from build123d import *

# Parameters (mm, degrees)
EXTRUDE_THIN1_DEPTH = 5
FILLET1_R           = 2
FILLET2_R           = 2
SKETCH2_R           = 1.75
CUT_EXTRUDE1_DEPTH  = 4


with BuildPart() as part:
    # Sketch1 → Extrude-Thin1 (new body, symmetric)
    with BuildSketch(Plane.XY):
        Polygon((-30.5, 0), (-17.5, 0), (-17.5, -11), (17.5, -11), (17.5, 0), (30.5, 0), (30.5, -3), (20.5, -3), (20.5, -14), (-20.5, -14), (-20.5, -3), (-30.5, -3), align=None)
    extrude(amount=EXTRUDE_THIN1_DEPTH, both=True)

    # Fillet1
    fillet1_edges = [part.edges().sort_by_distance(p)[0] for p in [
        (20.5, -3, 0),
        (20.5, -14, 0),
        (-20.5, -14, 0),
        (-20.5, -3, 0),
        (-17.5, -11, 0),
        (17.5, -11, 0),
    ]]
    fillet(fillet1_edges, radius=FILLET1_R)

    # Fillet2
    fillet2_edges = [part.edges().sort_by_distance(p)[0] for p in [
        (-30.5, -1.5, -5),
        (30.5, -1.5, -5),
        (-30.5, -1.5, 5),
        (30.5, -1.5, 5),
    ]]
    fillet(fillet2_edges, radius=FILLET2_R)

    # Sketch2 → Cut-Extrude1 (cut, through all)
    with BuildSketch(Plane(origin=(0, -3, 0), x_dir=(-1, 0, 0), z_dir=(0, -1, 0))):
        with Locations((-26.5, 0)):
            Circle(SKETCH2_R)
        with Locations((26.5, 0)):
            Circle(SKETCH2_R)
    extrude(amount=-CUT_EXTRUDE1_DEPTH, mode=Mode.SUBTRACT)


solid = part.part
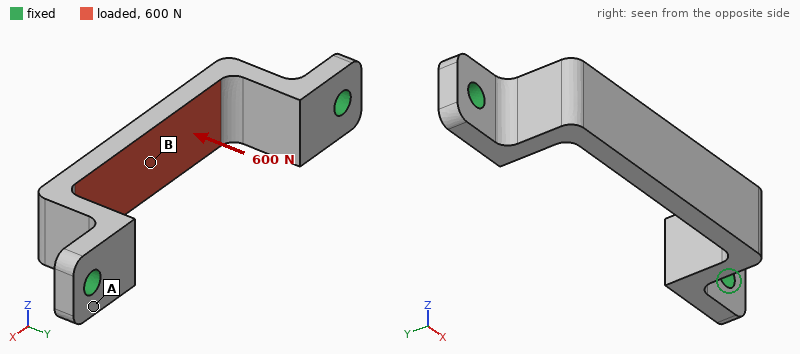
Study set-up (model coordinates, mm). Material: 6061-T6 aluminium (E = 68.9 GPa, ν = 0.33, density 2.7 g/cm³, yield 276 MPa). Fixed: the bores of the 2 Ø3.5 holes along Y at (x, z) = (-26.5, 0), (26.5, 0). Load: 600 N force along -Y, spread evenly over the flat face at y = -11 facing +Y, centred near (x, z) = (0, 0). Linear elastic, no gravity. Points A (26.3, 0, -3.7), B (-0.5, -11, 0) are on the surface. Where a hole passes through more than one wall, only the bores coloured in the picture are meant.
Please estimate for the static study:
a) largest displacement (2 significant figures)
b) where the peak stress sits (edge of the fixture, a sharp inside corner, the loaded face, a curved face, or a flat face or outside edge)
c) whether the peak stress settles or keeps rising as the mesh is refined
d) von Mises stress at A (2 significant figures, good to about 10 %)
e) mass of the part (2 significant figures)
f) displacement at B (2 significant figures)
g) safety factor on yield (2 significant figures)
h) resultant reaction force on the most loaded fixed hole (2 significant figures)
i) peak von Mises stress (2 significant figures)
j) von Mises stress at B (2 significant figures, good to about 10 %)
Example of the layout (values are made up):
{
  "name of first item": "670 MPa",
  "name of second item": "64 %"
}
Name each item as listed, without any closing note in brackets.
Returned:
{
  "largest displacement": "83 µm",
  "where the peak stress sits": "a curved face",
  "whether the peak stress settles or keeps rising as the mesh is refined": "settles",
  "von Mises stress at A": "18 MPa",
  "mass of the part": "6.6 g",
  "displacement at B": "80 µm",
  "safety factor on yield": "2.1",
  "resultant reaction force on the most loaded fixed hole": "430 N",
  "peak von Mises stress": "130 MPa",
  "von Mises stress at B": "65 MPa"
}
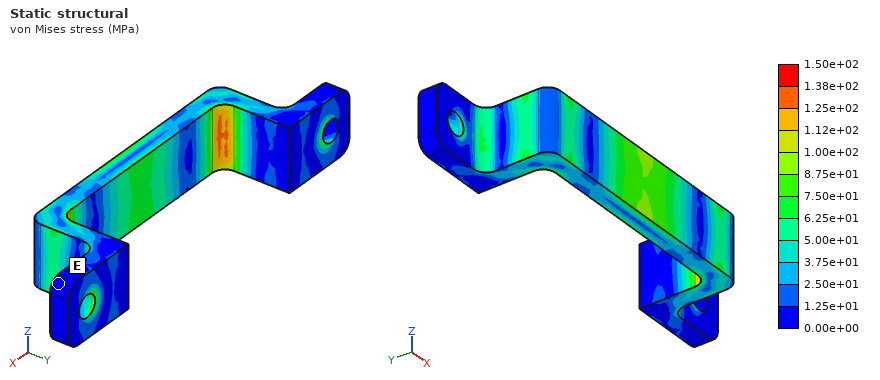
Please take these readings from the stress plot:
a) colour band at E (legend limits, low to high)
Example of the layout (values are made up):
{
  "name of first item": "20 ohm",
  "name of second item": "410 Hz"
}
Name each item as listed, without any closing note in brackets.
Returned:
{
  "colour band at E": "0.00e+00 to 1.25e+01 MPa"
}
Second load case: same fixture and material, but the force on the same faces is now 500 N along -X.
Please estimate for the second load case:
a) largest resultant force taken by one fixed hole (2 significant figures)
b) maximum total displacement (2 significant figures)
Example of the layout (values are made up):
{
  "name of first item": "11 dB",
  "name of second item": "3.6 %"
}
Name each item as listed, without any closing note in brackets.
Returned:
{
  "largest resultant force taken by one fixed hole": "260 N",
  "maximum total displacement": "61 µm"
}
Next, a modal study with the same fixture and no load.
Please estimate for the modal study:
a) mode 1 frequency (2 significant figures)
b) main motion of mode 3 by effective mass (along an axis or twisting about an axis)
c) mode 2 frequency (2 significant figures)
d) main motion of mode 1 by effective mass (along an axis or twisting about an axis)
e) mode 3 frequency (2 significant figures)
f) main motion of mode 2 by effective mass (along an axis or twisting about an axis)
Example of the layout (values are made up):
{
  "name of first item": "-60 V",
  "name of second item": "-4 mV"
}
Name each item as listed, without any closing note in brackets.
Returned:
{
  "mode 1 frequency": "6200 Hz",
  "main motion of mode 3 by effective mass": "along Y",
  "mode 2 frequency": "7500 Hz",
  "main motion of mode 1 by effective mass": "along Z",
  "mode 3 frequency": "9700 Hz",
  "main motion of mode 2 by effective mass": "along X"
}
